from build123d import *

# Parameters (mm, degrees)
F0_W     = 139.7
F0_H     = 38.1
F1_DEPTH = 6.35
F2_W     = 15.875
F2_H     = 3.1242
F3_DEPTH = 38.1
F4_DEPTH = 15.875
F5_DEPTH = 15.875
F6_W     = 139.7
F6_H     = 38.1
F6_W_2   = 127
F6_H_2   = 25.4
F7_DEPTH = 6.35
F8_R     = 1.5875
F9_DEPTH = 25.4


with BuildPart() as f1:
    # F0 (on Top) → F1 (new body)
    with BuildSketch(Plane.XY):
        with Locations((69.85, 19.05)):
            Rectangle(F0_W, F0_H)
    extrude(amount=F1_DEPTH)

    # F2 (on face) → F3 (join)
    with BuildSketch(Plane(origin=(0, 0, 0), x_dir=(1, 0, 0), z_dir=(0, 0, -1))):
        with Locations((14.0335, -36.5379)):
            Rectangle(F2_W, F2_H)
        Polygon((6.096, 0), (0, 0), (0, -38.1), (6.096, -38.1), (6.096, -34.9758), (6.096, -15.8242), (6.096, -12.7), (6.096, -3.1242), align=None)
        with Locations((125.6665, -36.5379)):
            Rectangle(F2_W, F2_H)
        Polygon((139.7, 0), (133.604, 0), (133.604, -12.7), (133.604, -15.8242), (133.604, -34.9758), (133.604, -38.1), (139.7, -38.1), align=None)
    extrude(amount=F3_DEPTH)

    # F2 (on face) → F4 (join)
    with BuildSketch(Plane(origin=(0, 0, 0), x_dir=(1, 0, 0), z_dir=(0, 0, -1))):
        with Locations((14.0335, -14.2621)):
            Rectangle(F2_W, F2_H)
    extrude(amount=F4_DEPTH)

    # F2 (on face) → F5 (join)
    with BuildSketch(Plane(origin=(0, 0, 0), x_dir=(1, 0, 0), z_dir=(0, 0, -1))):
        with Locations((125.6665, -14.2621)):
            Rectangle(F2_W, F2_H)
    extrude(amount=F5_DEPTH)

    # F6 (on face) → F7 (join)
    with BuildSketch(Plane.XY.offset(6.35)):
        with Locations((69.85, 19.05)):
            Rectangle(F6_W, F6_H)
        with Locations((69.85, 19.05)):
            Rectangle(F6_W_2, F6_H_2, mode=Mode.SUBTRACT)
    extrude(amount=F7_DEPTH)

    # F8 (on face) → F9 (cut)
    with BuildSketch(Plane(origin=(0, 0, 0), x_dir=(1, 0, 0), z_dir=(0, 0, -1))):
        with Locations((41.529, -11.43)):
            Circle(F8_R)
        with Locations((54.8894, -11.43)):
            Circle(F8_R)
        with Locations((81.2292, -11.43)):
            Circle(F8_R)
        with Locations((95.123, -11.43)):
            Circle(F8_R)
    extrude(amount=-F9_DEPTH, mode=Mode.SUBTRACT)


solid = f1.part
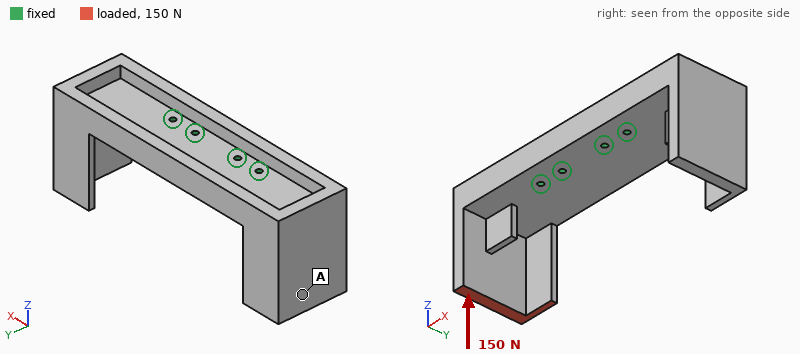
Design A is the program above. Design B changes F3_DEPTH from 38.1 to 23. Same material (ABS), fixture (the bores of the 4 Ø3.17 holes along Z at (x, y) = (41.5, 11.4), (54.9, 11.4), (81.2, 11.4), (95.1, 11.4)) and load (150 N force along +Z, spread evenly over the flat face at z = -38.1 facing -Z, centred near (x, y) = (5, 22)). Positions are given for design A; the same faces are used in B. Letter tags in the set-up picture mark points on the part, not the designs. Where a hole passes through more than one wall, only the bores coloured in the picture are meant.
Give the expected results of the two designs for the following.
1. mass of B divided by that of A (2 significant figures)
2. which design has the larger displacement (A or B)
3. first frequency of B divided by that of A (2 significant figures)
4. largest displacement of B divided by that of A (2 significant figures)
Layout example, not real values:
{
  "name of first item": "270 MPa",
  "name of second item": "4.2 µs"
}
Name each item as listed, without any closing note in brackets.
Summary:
{
  "mass of B divided by that of A": "0.88",
  "which design has the larger displacement": "A",
  "first frequency of B divided by that of A": "1.3",
  "largest displacement of B divided by that of A": "0.84"
}
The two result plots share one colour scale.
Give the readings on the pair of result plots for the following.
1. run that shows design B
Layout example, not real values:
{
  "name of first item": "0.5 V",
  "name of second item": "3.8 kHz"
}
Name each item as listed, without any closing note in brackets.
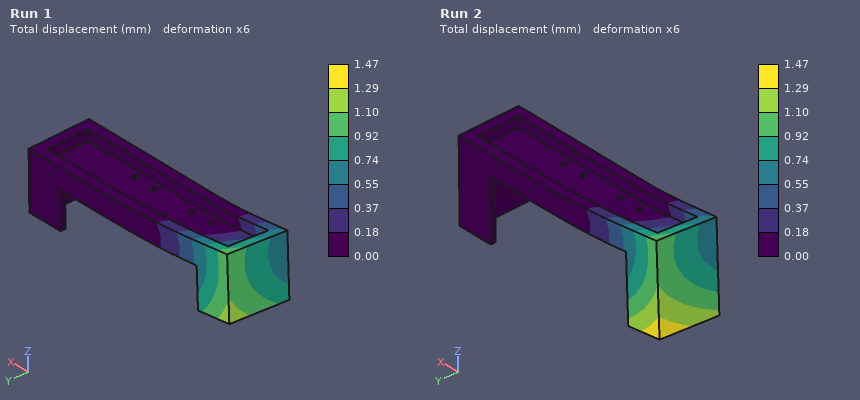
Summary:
{
  "run that shows design B": "Run 1"
}
